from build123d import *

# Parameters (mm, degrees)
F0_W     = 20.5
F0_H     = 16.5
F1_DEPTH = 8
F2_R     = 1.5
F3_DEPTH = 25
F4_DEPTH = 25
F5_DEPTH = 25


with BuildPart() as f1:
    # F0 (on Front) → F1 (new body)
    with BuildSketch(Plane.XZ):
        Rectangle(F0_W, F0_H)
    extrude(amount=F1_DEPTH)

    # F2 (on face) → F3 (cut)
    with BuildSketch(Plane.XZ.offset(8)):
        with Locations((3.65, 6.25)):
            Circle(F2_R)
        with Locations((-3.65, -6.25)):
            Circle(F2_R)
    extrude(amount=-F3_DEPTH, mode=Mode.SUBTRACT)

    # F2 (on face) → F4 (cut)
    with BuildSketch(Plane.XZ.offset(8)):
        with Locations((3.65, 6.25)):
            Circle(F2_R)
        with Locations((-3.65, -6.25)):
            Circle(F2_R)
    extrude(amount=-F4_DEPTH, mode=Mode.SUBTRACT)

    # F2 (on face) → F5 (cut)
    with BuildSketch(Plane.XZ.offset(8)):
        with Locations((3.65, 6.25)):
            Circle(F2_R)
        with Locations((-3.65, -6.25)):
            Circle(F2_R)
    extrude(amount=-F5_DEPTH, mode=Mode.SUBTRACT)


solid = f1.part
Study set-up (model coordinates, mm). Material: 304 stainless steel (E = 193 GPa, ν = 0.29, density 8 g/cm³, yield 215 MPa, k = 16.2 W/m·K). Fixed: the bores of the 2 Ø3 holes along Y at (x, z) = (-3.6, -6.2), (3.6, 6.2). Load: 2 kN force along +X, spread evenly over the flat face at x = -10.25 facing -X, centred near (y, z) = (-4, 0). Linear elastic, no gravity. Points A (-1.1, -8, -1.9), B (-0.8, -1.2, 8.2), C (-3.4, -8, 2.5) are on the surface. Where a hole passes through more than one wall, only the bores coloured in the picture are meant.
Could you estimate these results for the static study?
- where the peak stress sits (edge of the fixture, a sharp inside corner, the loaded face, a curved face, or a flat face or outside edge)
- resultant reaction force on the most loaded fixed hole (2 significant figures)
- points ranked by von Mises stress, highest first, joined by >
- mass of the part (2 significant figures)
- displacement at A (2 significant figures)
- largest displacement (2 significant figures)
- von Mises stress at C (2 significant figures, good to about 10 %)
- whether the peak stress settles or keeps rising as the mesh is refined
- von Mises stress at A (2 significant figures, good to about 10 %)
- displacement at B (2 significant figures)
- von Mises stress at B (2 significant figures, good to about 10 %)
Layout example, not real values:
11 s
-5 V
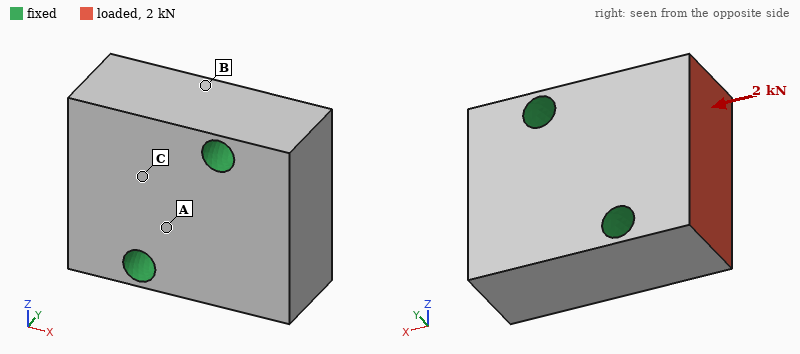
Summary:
edge of the fixture
1.0 kN
B > C > A
21 g
0.32 µm
1.4 µm
13 MPa
keeps rising
6.8 MPa
0.43 µm
21 MPa
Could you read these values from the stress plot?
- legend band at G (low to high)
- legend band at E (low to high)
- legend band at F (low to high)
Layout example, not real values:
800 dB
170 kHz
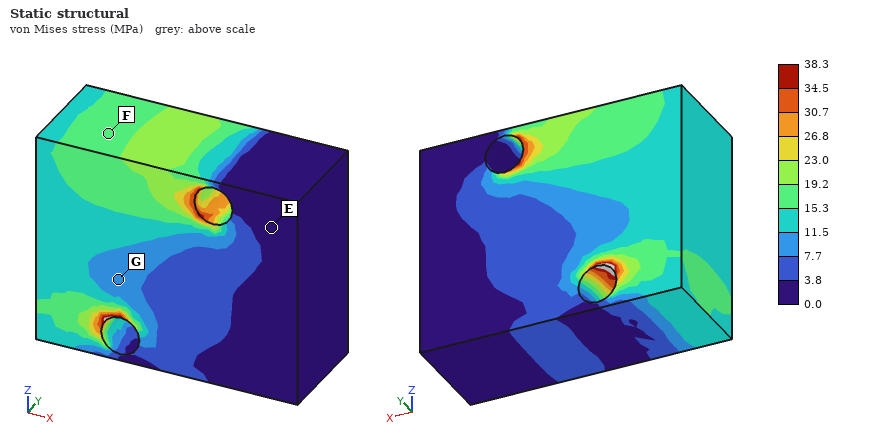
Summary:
7.7 to 11.5 MPa
0.0 to 3.8 MPa
15.3 to 19.2 MPa
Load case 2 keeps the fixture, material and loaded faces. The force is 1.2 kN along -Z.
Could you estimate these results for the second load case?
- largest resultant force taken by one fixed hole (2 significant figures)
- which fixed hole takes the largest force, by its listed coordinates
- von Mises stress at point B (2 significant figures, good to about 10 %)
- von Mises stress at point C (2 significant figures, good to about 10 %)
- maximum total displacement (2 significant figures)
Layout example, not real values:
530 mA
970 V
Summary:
1.2 kN
(-3.6, -6.2)
19 MPa
11 MPa
2.2 µm
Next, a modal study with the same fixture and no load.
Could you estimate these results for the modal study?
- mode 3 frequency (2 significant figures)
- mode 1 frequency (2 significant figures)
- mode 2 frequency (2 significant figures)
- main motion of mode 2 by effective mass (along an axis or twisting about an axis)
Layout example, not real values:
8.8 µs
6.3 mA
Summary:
70 kHz
38 kHz
45 kHz
along Y
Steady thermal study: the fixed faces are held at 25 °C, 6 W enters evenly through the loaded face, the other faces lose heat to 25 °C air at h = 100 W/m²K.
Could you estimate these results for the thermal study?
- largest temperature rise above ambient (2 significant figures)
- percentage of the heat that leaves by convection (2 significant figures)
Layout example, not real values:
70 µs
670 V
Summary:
27 K
11 %
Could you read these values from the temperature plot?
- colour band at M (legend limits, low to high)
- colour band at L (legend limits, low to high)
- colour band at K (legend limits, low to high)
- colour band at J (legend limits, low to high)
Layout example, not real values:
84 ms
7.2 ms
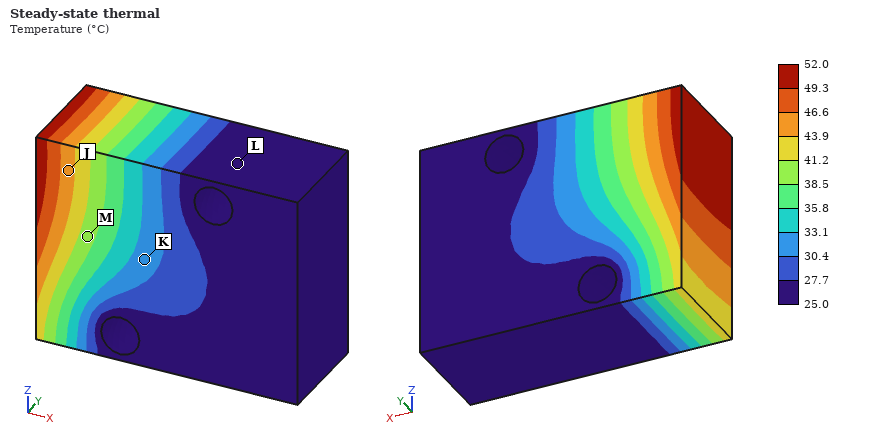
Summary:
38.5 to 41.2 °C
25.0 to 27.7 °C
30.4 to 33.1 °C
43.9 to 46.6 °C
